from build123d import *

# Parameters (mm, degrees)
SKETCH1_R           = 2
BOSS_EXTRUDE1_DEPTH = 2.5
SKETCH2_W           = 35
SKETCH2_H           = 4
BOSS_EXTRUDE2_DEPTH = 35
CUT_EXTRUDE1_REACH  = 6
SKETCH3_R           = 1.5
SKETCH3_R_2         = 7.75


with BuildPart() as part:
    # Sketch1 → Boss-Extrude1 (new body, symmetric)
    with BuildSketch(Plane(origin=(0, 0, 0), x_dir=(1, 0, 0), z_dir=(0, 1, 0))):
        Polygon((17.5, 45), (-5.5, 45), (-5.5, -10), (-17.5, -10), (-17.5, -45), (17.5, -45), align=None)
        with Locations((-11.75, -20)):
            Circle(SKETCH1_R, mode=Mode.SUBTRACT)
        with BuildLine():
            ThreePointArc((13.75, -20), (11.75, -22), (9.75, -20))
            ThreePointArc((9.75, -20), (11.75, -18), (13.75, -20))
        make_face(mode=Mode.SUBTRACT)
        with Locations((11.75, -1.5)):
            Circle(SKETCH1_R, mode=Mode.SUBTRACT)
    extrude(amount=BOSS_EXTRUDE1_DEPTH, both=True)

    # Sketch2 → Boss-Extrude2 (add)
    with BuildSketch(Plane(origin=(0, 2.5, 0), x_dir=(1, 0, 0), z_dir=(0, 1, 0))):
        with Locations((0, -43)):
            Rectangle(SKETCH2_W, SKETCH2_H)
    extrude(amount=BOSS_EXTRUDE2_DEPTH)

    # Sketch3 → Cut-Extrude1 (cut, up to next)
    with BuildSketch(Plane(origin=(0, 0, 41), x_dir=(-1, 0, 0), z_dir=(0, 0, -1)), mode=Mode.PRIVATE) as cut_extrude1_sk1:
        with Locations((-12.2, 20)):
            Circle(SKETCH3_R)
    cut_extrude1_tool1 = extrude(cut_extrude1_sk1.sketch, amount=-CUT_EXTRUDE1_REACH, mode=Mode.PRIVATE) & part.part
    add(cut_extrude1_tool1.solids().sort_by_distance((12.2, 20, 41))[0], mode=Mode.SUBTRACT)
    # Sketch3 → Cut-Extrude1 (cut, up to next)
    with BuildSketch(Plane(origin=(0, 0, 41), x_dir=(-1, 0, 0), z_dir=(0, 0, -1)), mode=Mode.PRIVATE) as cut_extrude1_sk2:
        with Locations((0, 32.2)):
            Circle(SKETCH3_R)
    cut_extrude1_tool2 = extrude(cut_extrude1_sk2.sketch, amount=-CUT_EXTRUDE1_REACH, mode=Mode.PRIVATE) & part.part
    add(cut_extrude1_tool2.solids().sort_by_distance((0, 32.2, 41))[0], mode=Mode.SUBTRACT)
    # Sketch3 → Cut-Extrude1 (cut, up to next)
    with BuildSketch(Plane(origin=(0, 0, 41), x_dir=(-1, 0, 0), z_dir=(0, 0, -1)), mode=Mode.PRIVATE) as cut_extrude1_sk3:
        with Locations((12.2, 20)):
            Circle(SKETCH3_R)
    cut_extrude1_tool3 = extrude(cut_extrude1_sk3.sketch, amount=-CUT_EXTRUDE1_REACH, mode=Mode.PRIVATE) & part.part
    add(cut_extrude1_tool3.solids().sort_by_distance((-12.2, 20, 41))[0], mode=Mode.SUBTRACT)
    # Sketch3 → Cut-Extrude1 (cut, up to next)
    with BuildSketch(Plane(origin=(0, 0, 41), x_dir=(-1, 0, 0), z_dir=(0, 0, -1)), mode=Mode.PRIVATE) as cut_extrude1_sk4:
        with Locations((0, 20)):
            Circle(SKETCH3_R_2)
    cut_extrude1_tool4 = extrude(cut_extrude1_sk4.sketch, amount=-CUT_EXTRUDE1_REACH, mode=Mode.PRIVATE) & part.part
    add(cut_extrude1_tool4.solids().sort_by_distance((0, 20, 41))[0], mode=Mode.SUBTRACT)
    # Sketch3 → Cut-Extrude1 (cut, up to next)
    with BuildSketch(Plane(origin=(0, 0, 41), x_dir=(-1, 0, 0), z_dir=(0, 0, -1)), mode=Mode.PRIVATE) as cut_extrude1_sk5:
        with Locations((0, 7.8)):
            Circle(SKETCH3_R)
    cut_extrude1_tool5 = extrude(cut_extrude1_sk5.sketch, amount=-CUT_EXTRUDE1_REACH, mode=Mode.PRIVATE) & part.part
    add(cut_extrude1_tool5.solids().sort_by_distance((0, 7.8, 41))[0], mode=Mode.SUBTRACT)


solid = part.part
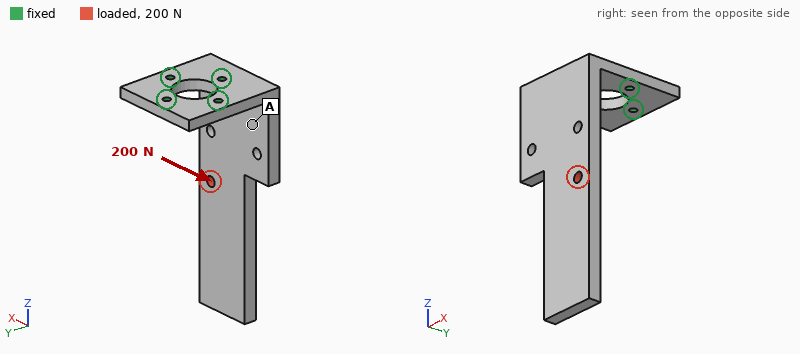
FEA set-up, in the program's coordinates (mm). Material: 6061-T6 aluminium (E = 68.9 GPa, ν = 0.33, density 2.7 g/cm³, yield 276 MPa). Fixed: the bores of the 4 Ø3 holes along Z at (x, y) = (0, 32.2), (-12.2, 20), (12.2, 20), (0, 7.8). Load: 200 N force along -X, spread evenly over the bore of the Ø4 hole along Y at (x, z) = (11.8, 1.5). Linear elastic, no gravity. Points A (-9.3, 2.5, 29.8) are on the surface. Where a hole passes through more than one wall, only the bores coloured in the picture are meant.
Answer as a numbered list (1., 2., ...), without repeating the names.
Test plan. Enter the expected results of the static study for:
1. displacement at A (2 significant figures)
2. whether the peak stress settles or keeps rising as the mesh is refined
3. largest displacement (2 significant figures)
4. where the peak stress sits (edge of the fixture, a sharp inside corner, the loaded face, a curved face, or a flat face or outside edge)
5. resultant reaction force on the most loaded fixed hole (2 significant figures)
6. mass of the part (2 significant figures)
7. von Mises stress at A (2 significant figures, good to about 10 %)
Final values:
1. 0.048 mm
2. keeps rising
3. 0.27 mm
4. edge of the fixture
5. 170 N
6. 44 g
7. 12 MPa
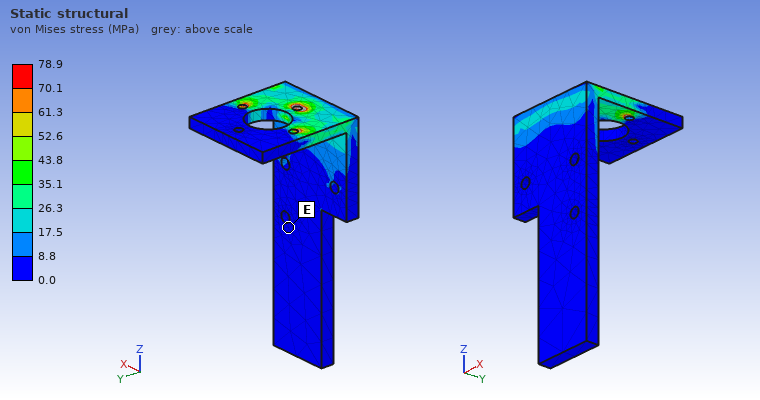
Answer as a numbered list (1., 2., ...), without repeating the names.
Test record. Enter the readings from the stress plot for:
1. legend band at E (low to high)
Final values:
1. 0.0 to 8.8 MPa
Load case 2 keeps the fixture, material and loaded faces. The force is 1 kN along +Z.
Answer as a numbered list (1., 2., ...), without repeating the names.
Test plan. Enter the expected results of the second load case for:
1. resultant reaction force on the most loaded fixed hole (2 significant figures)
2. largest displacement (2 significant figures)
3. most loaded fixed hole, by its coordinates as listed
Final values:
1. 1.2 kN
2. 0.52 mm
3. (0, 7.8)
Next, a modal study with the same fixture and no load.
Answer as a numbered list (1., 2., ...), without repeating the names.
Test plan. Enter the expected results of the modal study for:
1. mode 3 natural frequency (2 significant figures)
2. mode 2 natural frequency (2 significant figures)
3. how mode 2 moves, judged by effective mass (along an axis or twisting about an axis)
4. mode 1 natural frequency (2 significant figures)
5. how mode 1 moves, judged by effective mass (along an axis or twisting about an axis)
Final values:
1. 2700 Hz
2. 960 Hz
3. along X
4. 480 Hz
5. along Y
